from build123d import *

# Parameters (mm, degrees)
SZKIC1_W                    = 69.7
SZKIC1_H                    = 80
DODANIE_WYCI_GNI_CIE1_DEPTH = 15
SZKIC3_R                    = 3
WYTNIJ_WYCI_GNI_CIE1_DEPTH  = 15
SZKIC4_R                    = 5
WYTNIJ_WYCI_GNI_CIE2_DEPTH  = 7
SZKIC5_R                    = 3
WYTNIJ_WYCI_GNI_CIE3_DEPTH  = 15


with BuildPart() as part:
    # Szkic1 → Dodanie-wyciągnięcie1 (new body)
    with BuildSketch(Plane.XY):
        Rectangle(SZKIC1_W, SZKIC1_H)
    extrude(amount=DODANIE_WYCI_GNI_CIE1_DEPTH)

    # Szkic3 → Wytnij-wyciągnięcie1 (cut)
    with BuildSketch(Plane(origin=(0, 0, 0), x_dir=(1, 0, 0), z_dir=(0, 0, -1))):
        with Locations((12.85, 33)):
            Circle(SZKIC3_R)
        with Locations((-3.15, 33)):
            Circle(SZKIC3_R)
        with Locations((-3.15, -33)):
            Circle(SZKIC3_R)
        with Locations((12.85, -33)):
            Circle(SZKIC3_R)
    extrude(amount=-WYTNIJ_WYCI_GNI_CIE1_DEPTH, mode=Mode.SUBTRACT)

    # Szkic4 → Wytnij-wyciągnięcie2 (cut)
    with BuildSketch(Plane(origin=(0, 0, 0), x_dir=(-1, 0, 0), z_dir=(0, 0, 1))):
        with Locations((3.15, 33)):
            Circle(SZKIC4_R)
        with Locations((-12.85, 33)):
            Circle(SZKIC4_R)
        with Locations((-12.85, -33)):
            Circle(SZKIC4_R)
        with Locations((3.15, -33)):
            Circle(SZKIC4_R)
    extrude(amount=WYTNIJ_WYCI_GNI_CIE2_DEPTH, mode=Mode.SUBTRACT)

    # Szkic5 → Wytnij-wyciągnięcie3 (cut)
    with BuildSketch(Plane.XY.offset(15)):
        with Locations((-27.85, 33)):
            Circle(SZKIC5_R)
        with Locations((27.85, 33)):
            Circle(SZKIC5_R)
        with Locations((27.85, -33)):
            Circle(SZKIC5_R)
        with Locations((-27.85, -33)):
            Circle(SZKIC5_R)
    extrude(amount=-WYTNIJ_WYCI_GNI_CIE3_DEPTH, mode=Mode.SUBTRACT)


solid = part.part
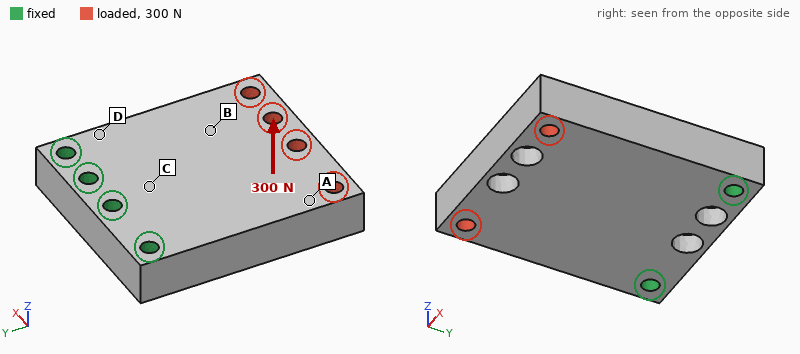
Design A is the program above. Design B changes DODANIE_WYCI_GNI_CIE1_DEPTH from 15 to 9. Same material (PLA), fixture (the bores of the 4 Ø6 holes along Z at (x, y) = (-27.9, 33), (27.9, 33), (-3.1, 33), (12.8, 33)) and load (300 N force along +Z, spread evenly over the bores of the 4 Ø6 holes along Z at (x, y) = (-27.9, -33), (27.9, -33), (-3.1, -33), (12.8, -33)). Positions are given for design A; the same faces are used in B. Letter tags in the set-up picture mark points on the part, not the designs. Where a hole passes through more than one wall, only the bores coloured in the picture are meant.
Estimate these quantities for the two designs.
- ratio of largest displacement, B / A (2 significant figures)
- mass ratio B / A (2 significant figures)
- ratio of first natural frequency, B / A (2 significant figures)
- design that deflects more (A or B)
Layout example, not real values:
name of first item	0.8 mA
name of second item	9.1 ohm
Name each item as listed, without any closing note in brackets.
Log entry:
ratio of largest displacement, B / A	4.4
mass ratio B / A	0.59
ratio of first natural frequency, B / A	0.62
design that deflects more	B
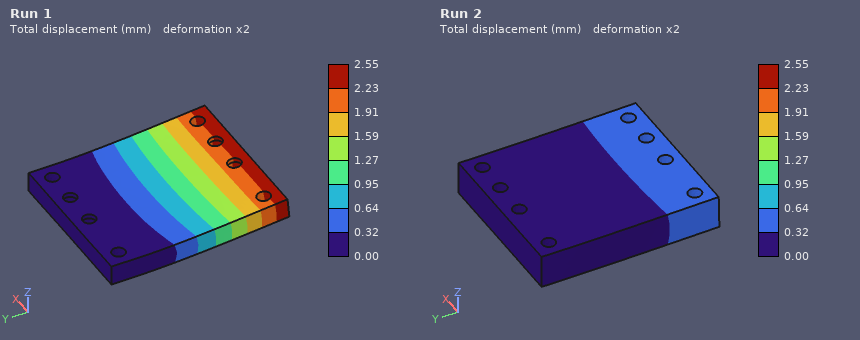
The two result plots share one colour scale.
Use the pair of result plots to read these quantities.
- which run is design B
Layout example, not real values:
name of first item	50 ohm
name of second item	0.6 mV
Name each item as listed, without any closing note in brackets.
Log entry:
which run is design B	Run 1
